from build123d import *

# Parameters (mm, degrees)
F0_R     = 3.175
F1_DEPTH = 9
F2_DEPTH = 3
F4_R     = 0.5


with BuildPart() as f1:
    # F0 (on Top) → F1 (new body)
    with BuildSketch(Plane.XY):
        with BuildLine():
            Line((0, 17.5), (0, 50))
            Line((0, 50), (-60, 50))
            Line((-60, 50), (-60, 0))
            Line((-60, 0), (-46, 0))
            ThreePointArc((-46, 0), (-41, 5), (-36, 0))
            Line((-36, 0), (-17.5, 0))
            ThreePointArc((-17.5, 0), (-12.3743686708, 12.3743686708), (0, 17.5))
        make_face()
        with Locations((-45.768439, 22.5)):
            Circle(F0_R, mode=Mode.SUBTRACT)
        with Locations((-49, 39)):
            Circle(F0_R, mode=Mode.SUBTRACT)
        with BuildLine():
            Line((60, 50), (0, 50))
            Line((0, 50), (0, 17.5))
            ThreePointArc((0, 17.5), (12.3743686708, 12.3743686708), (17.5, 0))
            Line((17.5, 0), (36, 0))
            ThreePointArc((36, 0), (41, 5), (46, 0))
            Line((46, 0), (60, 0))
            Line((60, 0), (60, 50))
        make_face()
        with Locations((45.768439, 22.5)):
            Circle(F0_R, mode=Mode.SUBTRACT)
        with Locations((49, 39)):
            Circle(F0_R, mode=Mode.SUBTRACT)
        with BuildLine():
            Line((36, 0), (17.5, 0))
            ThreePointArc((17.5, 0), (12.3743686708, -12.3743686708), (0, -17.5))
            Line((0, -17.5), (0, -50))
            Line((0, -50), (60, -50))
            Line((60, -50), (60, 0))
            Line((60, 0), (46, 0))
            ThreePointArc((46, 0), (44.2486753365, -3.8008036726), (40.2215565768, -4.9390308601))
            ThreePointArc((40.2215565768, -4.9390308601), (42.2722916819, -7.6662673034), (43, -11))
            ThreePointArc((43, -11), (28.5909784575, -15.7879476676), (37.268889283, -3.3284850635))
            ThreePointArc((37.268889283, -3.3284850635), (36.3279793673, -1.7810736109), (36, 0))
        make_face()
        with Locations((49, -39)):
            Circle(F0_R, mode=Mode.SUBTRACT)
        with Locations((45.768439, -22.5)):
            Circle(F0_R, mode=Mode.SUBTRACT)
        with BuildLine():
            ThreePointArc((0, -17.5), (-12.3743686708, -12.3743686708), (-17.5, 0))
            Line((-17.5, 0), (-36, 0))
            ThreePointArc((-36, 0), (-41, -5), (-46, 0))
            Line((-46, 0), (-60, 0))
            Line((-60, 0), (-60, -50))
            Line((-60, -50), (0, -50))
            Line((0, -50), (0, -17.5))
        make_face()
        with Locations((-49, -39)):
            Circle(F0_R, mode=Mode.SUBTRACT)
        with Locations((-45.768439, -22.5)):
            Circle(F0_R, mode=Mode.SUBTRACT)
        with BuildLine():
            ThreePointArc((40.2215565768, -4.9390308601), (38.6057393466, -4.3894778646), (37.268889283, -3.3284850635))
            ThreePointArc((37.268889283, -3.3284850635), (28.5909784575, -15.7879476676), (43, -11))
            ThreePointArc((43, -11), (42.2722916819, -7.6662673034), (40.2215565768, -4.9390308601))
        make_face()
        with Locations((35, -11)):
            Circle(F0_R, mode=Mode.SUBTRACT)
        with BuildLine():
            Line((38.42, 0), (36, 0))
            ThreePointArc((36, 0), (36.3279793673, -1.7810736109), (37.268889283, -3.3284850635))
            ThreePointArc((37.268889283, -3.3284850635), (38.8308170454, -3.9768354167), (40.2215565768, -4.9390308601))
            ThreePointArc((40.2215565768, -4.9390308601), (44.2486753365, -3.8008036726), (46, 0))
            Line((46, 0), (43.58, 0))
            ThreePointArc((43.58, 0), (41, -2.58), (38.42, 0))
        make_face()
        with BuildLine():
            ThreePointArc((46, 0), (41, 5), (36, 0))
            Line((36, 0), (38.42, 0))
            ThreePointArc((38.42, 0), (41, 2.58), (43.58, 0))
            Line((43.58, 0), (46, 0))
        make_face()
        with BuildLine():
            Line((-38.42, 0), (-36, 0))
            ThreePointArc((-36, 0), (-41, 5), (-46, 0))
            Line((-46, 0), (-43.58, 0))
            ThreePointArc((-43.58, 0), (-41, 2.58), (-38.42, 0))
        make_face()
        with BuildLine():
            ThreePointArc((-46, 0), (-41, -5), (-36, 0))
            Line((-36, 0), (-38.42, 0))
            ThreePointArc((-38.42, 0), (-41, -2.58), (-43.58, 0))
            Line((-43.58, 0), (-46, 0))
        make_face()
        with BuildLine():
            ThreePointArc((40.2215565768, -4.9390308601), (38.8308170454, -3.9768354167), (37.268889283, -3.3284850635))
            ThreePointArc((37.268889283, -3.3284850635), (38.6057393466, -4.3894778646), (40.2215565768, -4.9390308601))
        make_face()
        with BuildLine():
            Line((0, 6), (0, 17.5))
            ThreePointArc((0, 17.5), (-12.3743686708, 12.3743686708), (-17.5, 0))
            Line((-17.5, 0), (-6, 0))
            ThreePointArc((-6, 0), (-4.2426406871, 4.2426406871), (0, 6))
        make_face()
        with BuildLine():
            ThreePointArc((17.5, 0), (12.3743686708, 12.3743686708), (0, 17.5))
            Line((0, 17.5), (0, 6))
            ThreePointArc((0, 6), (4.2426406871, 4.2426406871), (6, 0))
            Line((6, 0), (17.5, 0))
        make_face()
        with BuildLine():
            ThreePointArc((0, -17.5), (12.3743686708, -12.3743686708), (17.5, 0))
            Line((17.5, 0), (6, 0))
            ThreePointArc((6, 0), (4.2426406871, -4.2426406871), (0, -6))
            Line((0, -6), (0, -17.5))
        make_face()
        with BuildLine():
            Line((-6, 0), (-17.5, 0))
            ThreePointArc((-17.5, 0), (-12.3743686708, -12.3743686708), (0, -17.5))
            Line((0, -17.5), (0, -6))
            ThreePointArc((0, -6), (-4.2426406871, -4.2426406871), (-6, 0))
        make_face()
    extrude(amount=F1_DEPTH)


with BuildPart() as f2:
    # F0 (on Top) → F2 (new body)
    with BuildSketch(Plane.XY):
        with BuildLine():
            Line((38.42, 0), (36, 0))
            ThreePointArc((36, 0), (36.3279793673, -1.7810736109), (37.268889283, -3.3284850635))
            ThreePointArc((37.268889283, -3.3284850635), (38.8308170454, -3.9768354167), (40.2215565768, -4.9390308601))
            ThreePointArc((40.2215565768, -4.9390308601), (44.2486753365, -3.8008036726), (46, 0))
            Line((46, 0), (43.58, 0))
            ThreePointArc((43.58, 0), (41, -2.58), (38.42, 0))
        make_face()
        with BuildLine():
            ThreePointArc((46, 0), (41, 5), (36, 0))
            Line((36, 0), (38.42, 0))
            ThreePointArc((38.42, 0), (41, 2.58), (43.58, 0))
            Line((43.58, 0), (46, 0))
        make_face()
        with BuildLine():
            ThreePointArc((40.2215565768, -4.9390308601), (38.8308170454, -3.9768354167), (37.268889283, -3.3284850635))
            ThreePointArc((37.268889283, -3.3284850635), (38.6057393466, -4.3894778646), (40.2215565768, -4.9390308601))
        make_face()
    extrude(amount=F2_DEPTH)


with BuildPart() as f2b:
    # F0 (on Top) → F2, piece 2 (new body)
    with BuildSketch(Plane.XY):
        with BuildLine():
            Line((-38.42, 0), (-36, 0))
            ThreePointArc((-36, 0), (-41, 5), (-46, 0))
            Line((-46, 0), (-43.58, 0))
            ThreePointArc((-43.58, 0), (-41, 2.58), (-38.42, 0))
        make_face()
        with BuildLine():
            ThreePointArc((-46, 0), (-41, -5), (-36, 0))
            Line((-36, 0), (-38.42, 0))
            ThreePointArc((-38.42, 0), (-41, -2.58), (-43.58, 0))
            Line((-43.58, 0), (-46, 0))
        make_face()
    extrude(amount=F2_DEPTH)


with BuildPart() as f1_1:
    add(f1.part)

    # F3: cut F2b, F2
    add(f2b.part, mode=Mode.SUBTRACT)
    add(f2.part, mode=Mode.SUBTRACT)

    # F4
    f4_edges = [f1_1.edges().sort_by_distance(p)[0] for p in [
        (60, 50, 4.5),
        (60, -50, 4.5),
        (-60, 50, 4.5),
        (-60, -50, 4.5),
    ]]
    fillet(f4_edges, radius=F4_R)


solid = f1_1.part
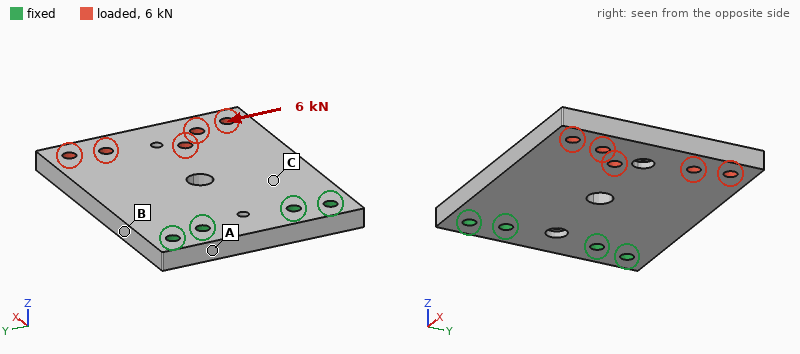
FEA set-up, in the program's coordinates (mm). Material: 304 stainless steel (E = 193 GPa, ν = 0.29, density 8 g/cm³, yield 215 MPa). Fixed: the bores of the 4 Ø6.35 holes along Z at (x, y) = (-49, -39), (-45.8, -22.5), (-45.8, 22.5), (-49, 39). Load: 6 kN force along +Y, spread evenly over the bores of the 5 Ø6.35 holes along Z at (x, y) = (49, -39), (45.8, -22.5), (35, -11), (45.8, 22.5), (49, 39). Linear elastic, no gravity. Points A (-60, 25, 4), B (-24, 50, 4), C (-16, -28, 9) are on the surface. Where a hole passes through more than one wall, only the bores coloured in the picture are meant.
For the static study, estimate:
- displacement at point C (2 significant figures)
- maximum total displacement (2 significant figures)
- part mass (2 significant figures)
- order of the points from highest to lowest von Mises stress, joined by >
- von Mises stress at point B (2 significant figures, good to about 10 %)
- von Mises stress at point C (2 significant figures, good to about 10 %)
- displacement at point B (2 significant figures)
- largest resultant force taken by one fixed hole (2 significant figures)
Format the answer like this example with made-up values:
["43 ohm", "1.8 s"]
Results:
["6.2 µm", "28 µm", "830 g", "B > C > A", "27 MPa", "18 MPa", "7.1 µm", "5.5 kN"]
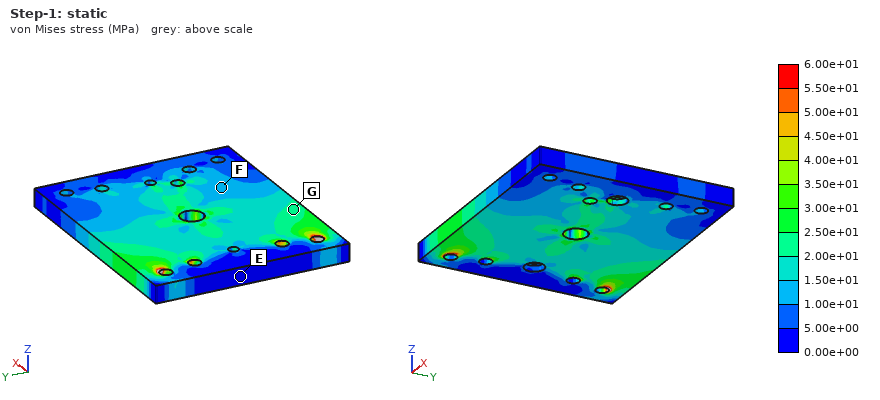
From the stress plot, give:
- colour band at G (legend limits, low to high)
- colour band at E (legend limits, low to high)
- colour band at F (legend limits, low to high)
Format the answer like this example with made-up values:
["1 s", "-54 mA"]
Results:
["2.00e+01 to 2.50e+01 MPa", "0.00e+00 to 5.00e+00 MPa", "1.00e+01 to 1.50e+01 MPa"]
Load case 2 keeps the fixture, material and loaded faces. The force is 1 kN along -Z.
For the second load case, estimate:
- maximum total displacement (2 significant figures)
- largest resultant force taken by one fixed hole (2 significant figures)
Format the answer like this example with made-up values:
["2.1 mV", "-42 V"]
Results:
["0.28 mm", "800 N"]
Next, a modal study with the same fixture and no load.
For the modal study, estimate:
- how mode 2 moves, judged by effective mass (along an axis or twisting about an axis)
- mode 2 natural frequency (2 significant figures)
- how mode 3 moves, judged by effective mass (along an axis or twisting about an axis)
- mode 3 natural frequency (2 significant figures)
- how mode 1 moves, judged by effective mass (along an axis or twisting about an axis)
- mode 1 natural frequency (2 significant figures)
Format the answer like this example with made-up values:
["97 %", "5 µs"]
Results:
["twisting about X", "1600 Hz", "along Z", "3700 Hz", "along Z", "630 Hz"]
